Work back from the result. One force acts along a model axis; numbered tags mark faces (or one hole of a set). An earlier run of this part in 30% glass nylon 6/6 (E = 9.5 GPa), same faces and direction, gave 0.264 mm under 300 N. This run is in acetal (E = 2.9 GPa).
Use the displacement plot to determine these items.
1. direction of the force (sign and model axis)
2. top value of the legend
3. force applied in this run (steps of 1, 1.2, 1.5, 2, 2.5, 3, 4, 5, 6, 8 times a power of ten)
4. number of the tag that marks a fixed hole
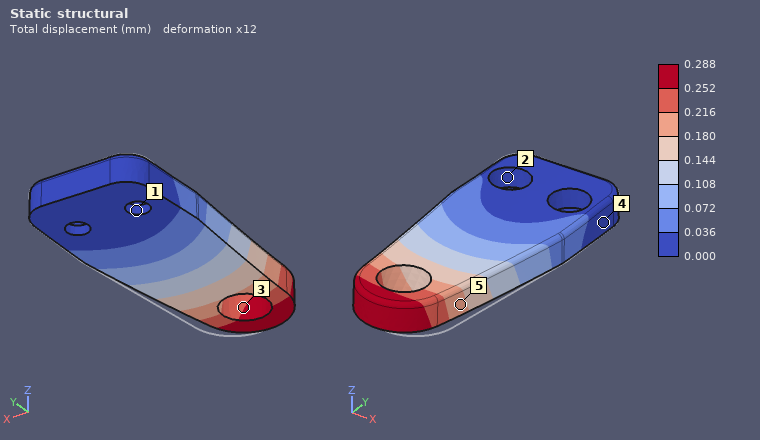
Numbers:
-X
0.288 mm
100 N
1
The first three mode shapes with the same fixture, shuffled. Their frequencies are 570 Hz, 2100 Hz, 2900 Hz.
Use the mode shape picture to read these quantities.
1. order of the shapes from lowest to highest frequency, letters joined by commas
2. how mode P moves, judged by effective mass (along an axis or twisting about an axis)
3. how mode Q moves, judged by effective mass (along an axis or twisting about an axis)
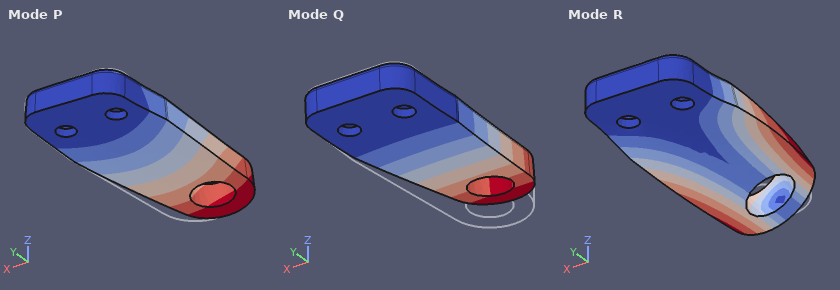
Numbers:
Q, P, R
along X
along Z
